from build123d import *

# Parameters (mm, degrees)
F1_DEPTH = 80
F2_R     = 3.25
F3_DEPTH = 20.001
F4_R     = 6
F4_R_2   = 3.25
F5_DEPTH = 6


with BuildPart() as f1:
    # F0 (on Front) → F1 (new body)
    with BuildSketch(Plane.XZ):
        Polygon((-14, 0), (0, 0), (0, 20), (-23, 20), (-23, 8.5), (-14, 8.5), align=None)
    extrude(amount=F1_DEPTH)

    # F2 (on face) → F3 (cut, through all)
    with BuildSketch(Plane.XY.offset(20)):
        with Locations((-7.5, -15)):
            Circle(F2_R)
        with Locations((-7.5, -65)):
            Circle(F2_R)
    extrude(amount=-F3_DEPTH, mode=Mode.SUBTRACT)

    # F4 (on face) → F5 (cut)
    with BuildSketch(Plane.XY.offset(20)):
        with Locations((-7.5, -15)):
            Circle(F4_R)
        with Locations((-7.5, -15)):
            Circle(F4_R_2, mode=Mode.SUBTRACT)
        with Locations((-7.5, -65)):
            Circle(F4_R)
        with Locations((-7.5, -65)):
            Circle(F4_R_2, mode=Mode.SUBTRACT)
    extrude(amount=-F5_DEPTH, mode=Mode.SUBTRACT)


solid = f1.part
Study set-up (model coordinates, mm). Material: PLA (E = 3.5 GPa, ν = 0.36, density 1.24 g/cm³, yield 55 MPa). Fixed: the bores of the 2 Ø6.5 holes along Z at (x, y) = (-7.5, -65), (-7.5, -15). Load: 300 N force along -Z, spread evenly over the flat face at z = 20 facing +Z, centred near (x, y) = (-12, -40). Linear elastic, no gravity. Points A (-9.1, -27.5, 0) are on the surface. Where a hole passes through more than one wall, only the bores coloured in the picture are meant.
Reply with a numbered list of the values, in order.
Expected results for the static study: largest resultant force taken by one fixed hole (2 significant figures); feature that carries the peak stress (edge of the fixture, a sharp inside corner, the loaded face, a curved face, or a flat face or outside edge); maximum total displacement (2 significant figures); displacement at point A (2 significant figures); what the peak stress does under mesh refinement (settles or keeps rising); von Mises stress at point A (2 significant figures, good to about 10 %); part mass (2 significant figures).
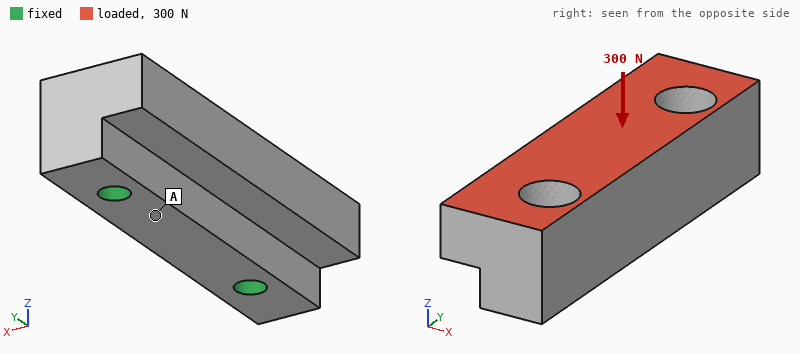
1. 150 N
2. edge of the fixture
3. 15 µm
4. 4.9 µm
5. keeps rising
6. 0.35 MPa
7. 35 g
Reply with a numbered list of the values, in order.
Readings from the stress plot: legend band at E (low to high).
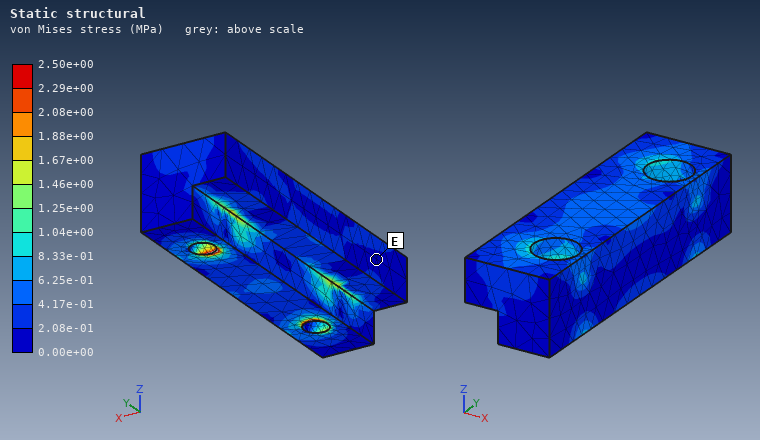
1. 0.00e+00 to 2.08e-01 MPa
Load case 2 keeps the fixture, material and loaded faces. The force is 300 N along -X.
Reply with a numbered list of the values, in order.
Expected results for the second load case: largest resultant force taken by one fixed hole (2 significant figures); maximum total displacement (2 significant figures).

1. 150 N
2. 29 µm
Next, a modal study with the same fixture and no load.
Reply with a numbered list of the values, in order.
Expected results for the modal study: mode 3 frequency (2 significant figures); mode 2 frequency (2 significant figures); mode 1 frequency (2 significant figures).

1. 7000 Hz
2. 6600 Hz
3. 5000 Hz
